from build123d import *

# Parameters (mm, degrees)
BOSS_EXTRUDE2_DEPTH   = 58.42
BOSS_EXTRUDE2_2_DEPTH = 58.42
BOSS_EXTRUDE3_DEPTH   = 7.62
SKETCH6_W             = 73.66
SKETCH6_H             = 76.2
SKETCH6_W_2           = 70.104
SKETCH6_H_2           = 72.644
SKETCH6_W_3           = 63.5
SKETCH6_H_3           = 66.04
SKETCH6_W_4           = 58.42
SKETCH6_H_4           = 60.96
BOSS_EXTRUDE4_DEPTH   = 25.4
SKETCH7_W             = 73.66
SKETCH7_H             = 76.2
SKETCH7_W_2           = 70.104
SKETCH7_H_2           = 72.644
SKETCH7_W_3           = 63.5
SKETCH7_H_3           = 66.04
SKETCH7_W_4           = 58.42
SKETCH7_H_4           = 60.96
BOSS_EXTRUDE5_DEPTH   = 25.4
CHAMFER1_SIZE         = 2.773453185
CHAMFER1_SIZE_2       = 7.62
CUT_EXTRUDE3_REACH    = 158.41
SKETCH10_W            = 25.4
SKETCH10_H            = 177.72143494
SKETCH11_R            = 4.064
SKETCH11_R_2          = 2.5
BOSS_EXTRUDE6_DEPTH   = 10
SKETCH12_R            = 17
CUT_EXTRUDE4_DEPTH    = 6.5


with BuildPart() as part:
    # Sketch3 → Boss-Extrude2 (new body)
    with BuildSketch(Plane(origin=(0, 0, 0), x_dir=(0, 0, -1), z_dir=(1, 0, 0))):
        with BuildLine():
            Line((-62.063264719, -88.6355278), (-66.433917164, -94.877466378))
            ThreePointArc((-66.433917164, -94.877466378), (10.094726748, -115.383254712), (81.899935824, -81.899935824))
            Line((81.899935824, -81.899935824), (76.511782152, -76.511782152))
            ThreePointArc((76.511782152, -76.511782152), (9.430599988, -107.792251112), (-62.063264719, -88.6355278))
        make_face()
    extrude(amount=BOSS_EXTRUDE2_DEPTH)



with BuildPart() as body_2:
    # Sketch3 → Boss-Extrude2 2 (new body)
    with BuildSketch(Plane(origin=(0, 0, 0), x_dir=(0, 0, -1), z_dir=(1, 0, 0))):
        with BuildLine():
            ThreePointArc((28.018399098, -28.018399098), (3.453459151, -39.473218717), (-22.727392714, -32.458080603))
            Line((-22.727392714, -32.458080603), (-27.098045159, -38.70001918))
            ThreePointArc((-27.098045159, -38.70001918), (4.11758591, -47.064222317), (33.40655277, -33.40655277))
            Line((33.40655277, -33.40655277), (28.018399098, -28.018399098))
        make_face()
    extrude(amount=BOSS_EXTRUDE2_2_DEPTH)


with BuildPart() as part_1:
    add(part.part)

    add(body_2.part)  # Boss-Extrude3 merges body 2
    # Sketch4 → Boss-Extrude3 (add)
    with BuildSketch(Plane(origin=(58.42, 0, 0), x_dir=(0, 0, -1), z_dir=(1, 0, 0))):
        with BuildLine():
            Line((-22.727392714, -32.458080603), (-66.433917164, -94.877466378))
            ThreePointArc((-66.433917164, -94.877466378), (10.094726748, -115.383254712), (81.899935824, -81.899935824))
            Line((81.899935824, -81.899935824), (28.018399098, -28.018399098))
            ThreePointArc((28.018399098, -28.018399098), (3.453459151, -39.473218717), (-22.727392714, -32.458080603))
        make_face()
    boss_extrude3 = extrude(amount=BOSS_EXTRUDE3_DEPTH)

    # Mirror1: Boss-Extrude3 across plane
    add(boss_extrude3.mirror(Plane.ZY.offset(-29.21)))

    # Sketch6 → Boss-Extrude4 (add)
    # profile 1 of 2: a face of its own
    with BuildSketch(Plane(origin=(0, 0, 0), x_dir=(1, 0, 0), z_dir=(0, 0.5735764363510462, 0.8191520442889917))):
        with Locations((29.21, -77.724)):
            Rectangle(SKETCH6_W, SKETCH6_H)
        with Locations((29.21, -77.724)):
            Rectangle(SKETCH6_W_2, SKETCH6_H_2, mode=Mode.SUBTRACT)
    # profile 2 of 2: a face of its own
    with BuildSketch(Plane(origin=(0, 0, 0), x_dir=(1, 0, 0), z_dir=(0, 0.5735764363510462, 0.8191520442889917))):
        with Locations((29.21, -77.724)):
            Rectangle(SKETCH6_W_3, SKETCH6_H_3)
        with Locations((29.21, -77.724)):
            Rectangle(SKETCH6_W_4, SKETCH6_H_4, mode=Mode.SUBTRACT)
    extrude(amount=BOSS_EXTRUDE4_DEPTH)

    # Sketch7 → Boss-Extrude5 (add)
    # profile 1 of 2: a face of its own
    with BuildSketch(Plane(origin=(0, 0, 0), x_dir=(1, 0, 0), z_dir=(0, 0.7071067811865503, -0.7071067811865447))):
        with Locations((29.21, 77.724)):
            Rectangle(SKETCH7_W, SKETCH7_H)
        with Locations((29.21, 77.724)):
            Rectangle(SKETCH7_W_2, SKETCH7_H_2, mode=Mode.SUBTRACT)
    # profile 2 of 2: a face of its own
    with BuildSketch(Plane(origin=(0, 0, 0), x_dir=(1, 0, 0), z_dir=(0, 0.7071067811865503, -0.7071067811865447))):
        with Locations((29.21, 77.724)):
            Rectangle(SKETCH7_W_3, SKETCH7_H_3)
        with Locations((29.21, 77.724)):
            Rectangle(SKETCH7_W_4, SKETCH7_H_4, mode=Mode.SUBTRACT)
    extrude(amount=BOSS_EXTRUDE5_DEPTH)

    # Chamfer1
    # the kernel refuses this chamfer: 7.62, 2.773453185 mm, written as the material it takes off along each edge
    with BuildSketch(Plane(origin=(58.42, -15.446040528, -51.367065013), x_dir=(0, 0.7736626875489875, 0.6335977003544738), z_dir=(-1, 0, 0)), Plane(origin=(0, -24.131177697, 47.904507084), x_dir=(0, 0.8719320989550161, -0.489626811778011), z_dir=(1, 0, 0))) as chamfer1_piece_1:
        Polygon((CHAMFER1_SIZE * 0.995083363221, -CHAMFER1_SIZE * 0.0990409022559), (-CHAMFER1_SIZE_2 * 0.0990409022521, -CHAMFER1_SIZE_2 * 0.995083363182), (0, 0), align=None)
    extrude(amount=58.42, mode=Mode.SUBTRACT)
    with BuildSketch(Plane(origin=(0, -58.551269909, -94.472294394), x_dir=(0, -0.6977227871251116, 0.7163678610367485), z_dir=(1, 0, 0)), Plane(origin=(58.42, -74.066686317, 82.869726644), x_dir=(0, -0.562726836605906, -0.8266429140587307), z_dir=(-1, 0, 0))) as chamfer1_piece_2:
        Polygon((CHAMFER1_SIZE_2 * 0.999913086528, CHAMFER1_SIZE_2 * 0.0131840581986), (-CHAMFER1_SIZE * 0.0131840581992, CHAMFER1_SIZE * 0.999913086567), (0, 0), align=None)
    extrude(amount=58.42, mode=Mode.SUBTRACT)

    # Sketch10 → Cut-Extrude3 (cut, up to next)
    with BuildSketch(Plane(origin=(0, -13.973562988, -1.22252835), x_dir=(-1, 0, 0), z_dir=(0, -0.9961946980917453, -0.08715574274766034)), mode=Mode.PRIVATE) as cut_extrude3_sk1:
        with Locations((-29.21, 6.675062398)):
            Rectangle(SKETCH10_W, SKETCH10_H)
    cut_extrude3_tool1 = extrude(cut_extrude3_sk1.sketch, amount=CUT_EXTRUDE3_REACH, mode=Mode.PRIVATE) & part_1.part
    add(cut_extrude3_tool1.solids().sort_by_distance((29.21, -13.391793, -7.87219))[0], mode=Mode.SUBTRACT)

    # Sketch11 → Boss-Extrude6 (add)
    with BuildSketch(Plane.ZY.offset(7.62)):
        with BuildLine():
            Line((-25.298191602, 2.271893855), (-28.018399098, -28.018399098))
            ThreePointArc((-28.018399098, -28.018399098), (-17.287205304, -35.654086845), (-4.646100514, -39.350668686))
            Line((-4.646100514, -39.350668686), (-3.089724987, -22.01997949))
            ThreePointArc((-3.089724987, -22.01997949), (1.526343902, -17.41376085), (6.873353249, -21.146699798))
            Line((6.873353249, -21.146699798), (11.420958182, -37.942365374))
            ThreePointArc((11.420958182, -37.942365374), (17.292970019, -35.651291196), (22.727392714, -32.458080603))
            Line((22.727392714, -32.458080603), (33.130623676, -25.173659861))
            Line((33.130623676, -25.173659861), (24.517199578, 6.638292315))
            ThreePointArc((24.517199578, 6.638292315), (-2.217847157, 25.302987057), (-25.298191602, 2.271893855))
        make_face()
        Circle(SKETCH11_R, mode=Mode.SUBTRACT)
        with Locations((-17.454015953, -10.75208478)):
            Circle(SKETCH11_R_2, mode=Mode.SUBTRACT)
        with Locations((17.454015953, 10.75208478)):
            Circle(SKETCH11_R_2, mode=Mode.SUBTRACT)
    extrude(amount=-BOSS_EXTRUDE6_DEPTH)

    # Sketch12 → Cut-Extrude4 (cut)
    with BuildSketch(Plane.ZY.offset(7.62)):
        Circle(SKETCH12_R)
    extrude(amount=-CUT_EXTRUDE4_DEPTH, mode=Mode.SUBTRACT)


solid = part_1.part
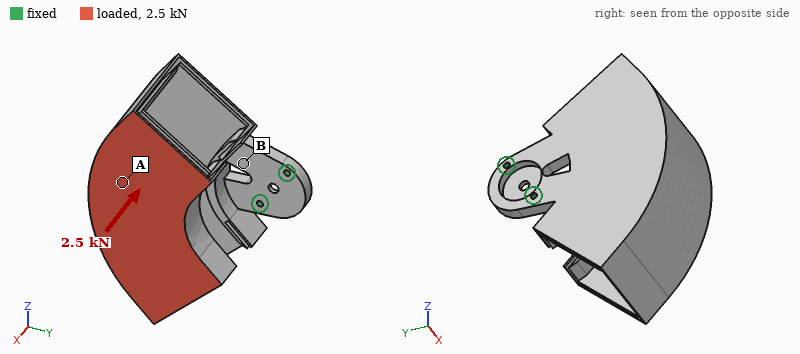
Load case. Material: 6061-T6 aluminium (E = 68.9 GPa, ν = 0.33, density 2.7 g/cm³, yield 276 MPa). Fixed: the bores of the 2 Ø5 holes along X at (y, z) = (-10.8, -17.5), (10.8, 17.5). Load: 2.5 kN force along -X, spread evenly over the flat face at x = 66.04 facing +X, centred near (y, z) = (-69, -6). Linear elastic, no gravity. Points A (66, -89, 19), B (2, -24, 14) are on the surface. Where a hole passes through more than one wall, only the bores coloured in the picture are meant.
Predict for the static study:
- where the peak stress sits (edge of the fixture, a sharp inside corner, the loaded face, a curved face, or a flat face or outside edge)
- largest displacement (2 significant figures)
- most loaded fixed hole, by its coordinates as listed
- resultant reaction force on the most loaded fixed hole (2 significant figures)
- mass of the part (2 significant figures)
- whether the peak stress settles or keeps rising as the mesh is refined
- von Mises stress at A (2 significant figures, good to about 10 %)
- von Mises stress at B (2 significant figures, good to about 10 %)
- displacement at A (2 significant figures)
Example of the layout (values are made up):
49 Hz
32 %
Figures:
edge of the fixture
2.1 mm
(-10.8, -17.5)
2.9 kN
770 g
keeps rising
30 MPa
110 MPa
1.9 mm
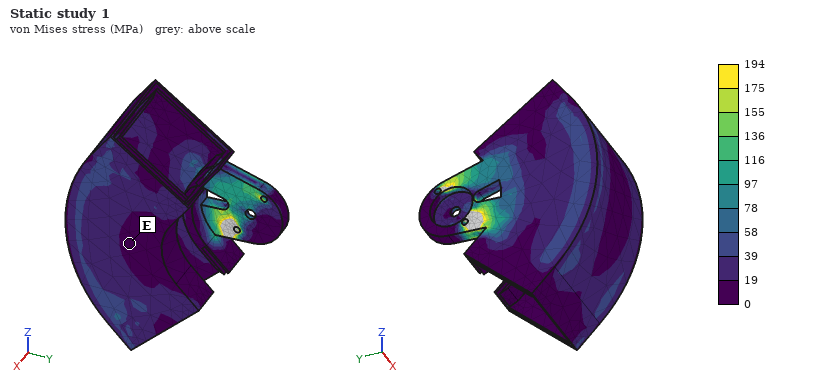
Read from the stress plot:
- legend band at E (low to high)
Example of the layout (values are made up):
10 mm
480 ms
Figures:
0 to 19 MPa
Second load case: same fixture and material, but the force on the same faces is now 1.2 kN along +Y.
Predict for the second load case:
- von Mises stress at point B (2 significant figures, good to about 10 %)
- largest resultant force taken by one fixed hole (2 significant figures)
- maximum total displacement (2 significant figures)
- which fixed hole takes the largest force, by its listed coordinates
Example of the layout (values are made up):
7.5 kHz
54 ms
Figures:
88 MPa
940 N
2.8 mm
(-10.8, -17.5)
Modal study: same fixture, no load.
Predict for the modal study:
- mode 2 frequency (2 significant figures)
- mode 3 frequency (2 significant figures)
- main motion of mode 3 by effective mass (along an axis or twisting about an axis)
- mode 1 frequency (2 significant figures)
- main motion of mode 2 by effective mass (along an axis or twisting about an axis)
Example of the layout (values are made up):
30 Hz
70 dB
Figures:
230 Hz
400 Hz
along X
170 Hz
along Z
